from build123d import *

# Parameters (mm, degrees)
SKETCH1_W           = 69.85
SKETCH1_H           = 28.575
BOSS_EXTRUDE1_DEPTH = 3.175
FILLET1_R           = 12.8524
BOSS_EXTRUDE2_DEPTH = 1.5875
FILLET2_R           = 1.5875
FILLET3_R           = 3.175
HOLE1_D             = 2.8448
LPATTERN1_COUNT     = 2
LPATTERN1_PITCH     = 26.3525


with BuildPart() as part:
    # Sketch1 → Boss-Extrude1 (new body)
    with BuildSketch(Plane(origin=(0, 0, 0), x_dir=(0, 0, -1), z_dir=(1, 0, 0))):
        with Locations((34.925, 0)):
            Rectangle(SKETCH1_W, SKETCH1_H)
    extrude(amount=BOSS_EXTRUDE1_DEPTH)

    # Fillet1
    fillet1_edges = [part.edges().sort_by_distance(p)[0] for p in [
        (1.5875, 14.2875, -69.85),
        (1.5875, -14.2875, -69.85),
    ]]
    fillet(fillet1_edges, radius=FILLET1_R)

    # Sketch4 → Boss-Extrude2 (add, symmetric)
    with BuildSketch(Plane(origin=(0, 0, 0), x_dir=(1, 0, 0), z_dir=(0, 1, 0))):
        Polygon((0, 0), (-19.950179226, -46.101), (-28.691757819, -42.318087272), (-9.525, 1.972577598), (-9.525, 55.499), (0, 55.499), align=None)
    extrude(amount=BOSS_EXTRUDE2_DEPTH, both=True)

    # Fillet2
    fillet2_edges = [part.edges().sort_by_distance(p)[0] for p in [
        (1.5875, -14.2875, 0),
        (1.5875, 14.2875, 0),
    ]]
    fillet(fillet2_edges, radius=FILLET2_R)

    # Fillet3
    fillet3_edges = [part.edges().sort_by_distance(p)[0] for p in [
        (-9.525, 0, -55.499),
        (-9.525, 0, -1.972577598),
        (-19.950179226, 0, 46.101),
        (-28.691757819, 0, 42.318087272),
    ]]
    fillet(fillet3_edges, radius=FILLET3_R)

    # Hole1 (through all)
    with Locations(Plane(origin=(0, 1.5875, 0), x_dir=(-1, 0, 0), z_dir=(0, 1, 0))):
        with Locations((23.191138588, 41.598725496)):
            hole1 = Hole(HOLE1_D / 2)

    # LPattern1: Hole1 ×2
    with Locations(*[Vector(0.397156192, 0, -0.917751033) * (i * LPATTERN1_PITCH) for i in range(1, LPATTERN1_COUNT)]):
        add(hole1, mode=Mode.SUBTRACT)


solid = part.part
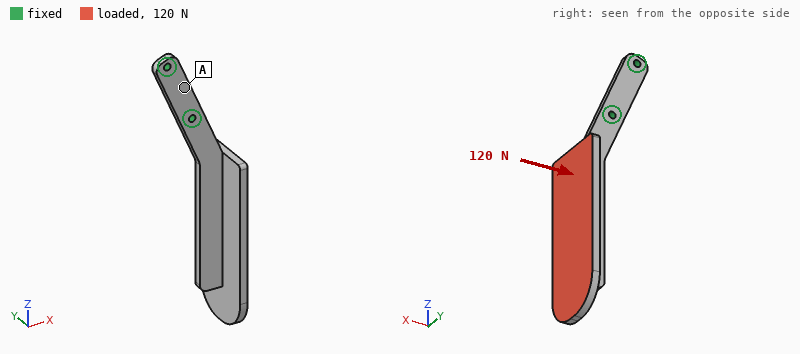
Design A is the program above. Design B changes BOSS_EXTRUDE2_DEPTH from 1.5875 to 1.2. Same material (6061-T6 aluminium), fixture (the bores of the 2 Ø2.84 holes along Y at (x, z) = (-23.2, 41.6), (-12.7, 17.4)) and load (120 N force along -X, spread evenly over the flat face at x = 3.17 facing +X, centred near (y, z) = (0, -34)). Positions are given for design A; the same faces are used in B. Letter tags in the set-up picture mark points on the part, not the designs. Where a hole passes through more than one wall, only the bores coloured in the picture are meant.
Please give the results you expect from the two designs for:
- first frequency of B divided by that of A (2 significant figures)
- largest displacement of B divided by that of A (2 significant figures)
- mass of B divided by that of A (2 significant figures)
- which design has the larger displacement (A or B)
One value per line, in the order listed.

0.68
1.3
0.92
B
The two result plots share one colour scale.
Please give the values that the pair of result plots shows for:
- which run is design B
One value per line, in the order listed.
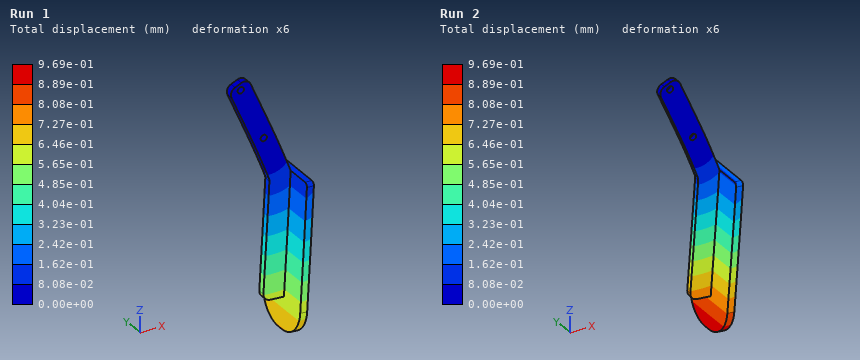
Run 2
